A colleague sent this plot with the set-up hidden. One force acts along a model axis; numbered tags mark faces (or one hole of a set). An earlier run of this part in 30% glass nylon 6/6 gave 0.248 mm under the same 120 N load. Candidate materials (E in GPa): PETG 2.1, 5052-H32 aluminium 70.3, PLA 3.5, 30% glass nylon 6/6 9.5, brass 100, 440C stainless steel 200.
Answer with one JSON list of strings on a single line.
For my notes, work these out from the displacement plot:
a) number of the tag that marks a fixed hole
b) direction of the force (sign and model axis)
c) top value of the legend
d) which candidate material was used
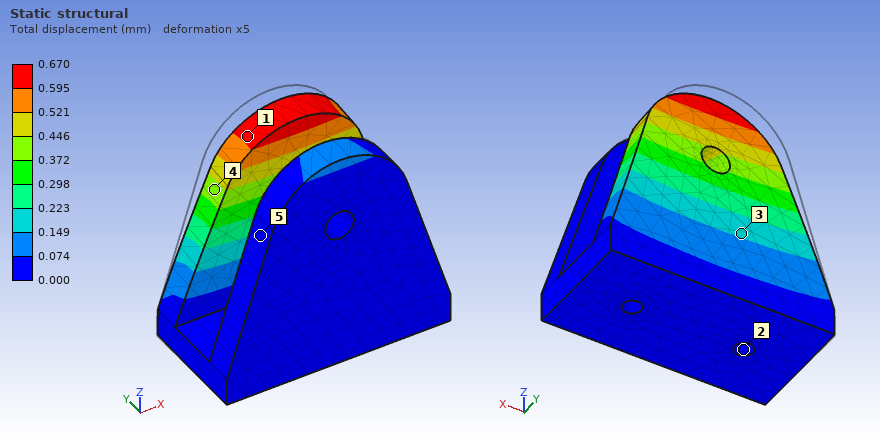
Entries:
["2", "-Y", "0.670 mm", "PLA"]
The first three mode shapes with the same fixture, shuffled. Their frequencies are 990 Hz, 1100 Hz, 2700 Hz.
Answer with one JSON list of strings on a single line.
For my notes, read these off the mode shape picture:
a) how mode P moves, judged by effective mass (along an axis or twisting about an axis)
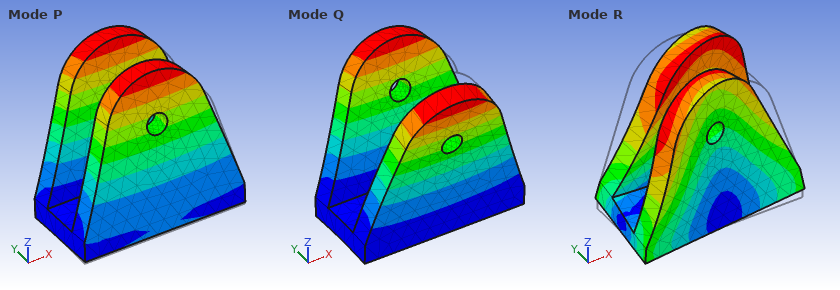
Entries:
["along Y"]
